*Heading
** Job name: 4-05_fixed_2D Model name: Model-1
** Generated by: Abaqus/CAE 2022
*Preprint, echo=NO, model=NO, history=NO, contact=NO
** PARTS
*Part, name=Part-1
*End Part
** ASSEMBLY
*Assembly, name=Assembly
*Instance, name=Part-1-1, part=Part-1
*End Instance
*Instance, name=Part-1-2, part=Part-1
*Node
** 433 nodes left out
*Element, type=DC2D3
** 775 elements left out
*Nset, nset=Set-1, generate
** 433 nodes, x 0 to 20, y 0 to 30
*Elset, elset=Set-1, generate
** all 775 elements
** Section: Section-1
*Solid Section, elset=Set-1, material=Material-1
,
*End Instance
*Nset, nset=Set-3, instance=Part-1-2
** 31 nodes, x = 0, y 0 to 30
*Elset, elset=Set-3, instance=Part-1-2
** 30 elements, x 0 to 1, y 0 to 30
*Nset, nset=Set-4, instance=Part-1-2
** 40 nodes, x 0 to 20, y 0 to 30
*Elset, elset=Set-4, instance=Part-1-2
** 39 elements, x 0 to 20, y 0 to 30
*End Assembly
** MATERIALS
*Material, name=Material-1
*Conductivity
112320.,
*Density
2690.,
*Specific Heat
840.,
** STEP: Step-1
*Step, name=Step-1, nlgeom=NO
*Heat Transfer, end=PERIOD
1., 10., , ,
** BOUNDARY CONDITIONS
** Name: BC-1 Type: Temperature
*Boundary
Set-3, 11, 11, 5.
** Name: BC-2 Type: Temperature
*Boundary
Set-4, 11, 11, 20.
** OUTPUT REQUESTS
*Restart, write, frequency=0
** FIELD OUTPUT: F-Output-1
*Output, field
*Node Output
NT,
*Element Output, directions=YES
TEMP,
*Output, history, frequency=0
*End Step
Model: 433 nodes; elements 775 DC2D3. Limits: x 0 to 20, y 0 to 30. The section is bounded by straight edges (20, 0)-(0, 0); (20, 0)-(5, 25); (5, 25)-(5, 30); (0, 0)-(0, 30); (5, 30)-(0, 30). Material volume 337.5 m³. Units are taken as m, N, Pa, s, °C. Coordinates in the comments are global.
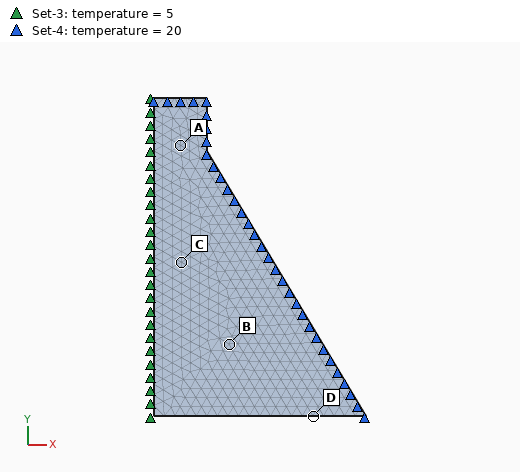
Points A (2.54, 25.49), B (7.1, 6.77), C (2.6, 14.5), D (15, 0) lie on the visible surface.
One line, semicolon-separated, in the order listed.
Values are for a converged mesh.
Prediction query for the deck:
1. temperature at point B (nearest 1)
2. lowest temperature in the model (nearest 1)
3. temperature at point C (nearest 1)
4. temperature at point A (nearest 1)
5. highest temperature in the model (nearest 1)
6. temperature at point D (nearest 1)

0 °C; 0 °C; 0 °C; 0 °C; 20 °C; 0 °C
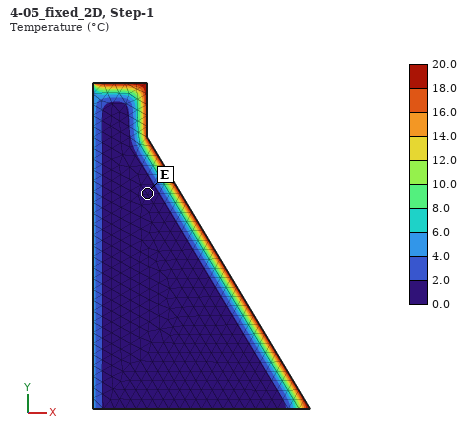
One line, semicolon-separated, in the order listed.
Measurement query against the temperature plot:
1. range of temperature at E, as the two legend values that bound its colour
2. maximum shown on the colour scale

0.0 to 2.0 °C; 20.0 °C
